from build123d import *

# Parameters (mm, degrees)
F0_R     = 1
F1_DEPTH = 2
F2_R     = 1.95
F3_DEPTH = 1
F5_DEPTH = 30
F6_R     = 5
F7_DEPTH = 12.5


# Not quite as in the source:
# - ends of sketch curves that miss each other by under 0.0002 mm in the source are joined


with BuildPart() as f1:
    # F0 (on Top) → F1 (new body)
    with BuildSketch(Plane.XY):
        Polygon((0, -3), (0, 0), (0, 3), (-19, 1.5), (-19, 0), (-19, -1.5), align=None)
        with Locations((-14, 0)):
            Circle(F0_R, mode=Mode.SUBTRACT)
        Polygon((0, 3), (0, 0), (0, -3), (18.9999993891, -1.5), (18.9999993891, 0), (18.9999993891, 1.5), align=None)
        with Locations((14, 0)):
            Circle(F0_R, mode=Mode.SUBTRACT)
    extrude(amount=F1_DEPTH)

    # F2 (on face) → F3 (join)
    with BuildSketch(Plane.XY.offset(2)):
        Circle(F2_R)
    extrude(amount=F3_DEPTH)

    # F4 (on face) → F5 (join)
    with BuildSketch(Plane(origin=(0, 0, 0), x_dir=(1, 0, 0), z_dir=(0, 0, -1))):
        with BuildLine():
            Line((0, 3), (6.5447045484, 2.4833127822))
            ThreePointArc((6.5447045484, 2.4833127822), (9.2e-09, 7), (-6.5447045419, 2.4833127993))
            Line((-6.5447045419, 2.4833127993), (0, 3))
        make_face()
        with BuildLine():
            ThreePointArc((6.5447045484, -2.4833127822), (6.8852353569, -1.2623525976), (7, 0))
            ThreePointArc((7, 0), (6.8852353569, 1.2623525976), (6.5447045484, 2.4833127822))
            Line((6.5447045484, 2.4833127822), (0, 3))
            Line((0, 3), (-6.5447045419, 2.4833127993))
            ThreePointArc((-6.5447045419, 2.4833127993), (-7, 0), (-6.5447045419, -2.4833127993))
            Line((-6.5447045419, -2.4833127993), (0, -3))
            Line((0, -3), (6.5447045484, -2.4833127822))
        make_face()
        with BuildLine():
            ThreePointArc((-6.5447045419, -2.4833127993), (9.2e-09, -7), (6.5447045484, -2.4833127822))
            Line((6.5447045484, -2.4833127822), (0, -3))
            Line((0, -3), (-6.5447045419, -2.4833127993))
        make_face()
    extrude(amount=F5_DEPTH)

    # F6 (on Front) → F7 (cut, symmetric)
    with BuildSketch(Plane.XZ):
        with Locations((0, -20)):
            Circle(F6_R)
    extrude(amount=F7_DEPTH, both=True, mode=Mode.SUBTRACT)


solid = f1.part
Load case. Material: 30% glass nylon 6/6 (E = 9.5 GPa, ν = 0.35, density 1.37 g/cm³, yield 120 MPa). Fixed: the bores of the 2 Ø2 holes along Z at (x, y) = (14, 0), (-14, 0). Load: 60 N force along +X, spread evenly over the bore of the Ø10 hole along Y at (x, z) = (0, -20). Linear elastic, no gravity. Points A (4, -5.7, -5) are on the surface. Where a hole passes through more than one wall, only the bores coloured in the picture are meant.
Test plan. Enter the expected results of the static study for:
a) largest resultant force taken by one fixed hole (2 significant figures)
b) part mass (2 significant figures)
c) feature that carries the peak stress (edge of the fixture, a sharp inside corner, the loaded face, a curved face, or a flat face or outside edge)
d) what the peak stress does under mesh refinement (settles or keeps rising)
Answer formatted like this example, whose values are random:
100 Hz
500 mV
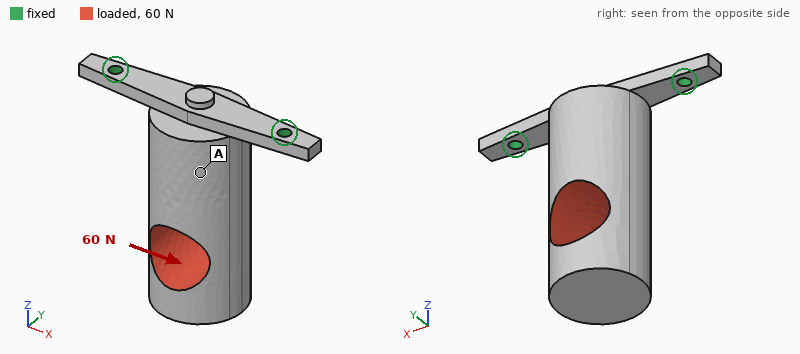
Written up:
68 N
5.4 g
edge of the fixture
keeps rising
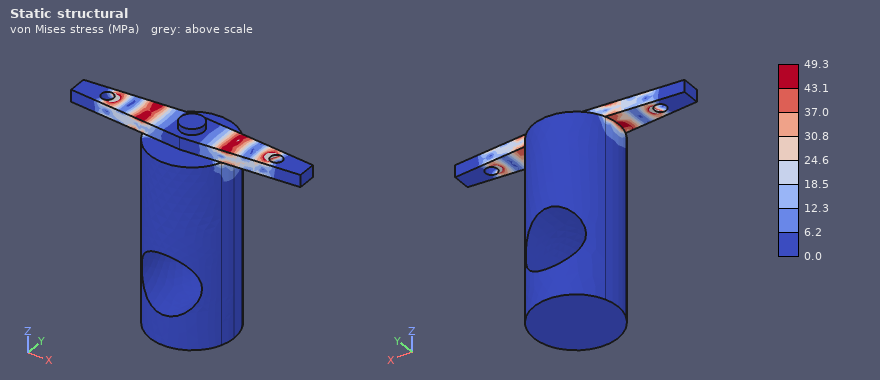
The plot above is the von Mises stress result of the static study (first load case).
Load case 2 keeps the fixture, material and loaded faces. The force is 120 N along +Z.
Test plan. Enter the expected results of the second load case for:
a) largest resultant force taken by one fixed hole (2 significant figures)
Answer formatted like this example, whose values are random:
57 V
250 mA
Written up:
68 N
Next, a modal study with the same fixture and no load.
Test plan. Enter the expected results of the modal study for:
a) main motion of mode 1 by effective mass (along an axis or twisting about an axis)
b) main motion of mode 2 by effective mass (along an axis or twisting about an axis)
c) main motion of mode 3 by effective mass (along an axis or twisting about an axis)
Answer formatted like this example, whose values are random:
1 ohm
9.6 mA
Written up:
along Y
along X
along Z
